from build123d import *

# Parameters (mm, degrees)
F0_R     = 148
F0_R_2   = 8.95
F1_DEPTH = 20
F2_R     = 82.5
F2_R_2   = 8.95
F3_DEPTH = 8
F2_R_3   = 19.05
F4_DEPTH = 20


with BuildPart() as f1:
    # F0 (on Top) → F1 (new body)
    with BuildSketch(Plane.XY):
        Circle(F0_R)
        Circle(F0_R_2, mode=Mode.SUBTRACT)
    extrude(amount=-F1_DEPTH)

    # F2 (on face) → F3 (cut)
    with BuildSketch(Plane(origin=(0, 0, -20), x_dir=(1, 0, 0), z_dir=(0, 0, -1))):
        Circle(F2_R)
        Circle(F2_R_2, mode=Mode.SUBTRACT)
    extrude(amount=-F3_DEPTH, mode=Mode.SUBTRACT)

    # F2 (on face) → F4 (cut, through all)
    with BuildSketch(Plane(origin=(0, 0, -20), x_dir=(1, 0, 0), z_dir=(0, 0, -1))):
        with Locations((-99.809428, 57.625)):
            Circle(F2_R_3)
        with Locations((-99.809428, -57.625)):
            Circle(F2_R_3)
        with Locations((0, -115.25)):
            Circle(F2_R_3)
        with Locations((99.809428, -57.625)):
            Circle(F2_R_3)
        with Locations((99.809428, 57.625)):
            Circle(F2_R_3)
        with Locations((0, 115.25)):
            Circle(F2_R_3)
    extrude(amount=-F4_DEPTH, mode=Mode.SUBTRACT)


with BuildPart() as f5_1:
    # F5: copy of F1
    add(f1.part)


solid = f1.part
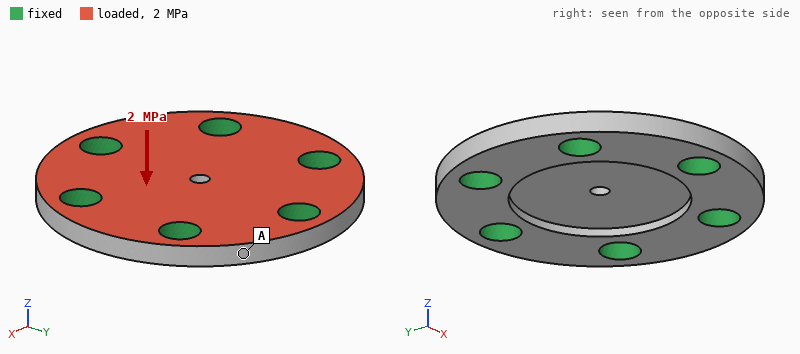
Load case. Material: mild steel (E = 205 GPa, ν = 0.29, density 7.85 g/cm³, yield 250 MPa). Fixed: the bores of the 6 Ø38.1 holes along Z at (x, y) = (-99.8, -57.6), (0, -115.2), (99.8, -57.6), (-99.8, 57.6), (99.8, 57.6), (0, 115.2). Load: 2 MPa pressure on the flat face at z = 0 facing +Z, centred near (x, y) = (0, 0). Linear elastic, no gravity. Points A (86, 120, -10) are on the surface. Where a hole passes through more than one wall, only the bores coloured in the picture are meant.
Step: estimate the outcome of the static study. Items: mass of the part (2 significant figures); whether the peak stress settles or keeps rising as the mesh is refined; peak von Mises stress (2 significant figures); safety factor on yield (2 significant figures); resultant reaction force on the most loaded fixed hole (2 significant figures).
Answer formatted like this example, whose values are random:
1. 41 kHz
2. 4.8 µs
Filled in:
1. 8.4 kg
2. settles
3. 110 MPa
4. 2.3
5. 21 kN
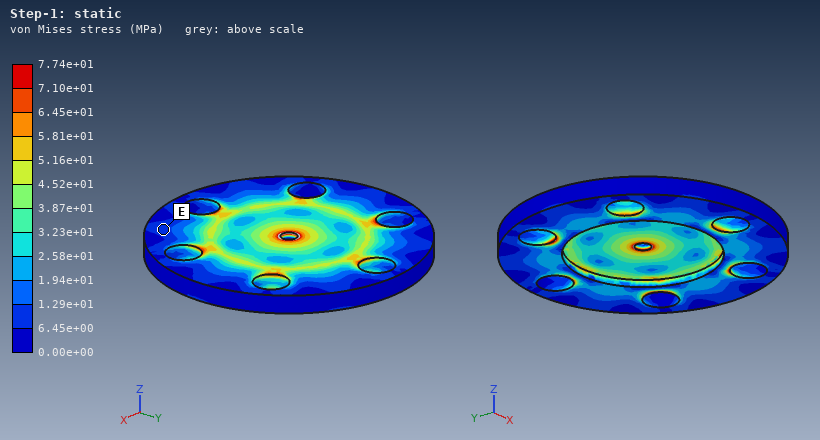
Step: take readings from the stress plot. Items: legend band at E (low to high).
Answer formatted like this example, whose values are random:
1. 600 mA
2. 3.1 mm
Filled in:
1. 6.45e+00 to 1.29e+01 MPa
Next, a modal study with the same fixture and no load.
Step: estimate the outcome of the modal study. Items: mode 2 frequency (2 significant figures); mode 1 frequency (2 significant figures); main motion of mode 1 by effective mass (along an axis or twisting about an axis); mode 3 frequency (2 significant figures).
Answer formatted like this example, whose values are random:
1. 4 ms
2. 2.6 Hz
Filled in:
1. 6400 Hz
2. 3300 Hz
3. along Z
4. 6400 Hz
